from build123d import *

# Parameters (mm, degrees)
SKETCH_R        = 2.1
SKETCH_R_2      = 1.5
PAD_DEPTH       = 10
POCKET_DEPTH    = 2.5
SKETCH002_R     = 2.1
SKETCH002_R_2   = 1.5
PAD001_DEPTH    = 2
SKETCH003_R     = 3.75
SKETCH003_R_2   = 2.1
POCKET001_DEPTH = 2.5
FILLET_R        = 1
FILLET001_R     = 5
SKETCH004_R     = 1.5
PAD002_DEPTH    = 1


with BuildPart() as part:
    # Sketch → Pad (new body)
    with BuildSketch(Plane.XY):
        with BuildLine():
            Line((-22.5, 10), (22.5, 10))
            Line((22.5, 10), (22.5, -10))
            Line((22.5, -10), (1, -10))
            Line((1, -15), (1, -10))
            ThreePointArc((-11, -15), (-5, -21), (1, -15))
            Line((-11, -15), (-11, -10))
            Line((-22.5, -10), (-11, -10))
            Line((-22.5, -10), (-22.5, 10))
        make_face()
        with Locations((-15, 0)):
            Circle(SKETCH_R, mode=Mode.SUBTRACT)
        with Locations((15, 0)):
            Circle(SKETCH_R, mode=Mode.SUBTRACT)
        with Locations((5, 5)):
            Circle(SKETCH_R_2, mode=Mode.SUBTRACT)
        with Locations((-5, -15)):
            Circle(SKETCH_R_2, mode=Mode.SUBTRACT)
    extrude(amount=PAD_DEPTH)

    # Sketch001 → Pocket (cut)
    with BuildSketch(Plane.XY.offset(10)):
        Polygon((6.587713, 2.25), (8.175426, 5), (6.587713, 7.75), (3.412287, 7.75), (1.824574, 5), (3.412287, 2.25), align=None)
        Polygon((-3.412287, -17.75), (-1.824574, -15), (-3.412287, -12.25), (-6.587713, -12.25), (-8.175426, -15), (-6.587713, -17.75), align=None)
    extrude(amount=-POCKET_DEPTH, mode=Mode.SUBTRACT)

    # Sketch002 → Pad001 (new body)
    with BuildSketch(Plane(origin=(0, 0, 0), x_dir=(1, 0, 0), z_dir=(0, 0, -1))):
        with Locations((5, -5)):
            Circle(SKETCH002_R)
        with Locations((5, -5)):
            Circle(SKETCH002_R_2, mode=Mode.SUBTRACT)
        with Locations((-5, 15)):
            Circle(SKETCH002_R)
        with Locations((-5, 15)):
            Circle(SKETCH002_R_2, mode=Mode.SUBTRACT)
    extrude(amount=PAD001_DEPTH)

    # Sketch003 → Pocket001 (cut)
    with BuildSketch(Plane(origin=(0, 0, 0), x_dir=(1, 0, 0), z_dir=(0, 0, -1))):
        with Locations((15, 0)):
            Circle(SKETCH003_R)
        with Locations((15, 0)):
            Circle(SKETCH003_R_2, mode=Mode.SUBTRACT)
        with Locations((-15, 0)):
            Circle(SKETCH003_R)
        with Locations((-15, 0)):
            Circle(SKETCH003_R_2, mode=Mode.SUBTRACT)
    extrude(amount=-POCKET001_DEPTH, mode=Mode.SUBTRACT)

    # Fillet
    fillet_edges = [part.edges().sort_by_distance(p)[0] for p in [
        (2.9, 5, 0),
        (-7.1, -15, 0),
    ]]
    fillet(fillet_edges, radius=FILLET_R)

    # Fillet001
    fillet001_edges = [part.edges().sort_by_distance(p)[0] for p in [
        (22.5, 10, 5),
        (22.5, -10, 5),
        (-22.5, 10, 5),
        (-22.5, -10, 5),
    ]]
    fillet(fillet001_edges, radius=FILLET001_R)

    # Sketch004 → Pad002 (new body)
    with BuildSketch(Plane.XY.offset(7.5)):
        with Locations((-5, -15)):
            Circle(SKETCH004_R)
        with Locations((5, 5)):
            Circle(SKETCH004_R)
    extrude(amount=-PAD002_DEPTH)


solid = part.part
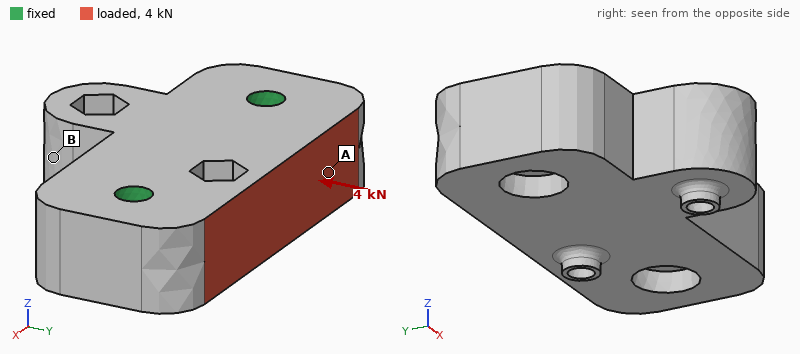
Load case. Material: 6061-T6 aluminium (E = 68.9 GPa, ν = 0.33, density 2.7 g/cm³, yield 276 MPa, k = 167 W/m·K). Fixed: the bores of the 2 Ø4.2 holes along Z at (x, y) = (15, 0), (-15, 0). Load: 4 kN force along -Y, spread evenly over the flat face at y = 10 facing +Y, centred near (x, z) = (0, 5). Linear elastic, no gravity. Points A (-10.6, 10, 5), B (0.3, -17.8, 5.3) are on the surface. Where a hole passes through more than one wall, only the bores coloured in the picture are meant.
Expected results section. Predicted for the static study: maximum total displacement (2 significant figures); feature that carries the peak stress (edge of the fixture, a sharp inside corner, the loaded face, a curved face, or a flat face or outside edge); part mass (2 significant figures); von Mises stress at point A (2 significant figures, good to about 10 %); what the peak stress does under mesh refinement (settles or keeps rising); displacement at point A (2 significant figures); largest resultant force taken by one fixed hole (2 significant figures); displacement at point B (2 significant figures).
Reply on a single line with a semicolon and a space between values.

7.5 µm; edge of the fixture; 25 g; 12 MPa; keeps rising; 4.4 µm; 2.0 kN; 5.8 µm
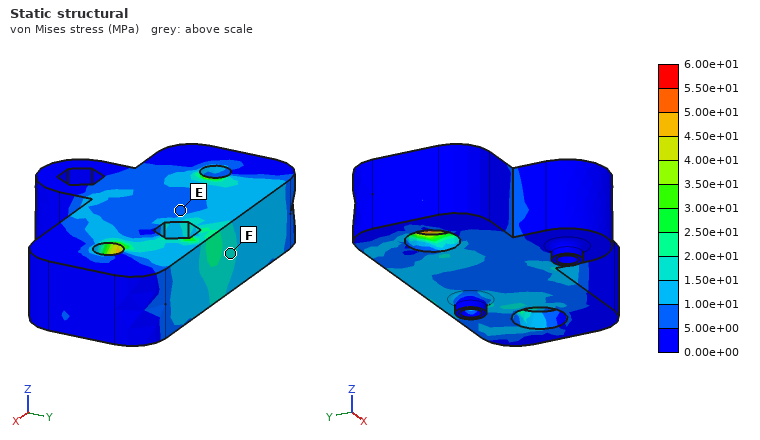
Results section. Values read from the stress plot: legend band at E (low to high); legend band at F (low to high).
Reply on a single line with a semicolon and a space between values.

5.00e+00 to 1.00e+01 MPa; 1.50e+01 to 2.00e+01 MPa
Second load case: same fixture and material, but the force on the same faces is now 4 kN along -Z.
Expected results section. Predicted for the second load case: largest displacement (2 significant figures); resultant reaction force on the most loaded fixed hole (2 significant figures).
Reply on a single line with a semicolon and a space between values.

37 µm; 2.0 kN
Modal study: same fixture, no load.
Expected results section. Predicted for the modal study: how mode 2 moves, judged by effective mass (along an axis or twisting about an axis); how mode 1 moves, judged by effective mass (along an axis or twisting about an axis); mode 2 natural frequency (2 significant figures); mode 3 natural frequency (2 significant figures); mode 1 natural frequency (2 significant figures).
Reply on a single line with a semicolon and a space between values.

along Z; along Z; 28 kHz; 30 kHz; 16 kHz
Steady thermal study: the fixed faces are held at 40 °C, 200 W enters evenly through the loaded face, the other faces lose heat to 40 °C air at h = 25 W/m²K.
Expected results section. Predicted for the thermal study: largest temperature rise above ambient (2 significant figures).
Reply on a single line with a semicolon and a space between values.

54 K
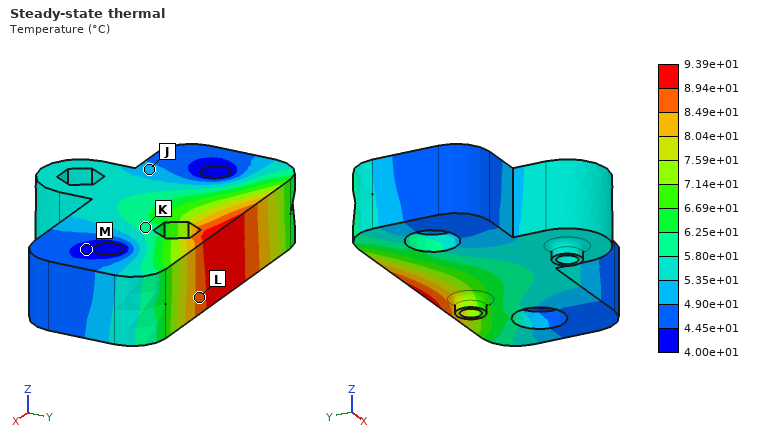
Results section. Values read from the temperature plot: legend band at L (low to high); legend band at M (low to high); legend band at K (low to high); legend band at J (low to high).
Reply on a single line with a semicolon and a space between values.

8.49e+01 to 8.94e+01 °C; 4.00e+01 to 4.45e+01 °C; 5.80e+01 to 6.25e+01 °C; 4.90e+01 to 5.35e+01 °C
